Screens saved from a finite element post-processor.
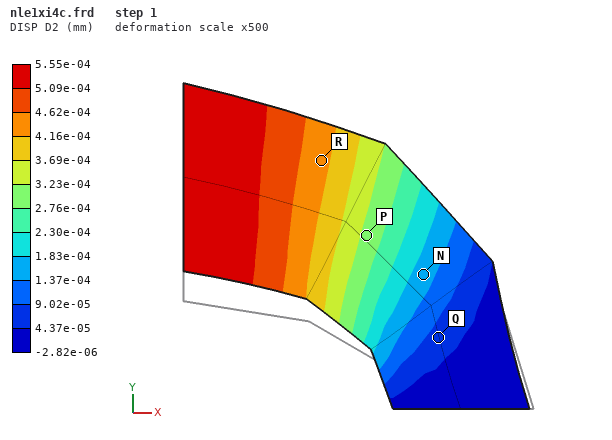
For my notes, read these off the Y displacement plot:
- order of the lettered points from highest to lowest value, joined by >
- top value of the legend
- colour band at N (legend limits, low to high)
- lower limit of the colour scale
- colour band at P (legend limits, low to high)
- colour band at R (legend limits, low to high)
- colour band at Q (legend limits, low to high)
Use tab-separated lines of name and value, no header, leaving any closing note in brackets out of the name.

order of the lettered points from highest to lowest value, joined by >	R > P > N > Q
top value of the legend	5.55e-04 mm
colour band at N	1.37e-04 to 1.83e-04 mm
lower limit of the colour scale	-2.82e-06 mm
colour band at P	2.76e-04 to 3.23e-04 mm
colour band at R	4.16e-04 to 4.62e-04 mm
colour band at Q	4.37e-05 to 9.02e-05 mm
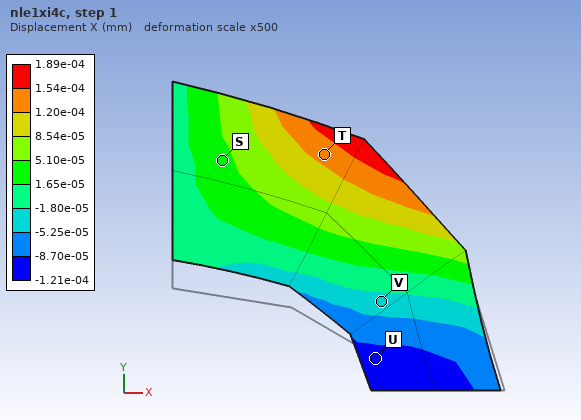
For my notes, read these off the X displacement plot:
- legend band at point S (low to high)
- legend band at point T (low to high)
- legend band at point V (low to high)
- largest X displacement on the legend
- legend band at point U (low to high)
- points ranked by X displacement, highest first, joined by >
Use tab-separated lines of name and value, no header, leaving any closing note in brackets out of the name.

legend band at point S	1.65e-05 to 5.10e-05 mm
legend band at point T	1.20e-04 to 1.54e-04 mm
legend band at point V	-5.25e-05 to -1.80e-05 mm
largest X displacement on the legend	1.89e-04 mm
legend band at point U	-1.21e-04 to -8.70e-05 mm
points ranked by X displacement, highest first, joined by >	T > S > V > U
